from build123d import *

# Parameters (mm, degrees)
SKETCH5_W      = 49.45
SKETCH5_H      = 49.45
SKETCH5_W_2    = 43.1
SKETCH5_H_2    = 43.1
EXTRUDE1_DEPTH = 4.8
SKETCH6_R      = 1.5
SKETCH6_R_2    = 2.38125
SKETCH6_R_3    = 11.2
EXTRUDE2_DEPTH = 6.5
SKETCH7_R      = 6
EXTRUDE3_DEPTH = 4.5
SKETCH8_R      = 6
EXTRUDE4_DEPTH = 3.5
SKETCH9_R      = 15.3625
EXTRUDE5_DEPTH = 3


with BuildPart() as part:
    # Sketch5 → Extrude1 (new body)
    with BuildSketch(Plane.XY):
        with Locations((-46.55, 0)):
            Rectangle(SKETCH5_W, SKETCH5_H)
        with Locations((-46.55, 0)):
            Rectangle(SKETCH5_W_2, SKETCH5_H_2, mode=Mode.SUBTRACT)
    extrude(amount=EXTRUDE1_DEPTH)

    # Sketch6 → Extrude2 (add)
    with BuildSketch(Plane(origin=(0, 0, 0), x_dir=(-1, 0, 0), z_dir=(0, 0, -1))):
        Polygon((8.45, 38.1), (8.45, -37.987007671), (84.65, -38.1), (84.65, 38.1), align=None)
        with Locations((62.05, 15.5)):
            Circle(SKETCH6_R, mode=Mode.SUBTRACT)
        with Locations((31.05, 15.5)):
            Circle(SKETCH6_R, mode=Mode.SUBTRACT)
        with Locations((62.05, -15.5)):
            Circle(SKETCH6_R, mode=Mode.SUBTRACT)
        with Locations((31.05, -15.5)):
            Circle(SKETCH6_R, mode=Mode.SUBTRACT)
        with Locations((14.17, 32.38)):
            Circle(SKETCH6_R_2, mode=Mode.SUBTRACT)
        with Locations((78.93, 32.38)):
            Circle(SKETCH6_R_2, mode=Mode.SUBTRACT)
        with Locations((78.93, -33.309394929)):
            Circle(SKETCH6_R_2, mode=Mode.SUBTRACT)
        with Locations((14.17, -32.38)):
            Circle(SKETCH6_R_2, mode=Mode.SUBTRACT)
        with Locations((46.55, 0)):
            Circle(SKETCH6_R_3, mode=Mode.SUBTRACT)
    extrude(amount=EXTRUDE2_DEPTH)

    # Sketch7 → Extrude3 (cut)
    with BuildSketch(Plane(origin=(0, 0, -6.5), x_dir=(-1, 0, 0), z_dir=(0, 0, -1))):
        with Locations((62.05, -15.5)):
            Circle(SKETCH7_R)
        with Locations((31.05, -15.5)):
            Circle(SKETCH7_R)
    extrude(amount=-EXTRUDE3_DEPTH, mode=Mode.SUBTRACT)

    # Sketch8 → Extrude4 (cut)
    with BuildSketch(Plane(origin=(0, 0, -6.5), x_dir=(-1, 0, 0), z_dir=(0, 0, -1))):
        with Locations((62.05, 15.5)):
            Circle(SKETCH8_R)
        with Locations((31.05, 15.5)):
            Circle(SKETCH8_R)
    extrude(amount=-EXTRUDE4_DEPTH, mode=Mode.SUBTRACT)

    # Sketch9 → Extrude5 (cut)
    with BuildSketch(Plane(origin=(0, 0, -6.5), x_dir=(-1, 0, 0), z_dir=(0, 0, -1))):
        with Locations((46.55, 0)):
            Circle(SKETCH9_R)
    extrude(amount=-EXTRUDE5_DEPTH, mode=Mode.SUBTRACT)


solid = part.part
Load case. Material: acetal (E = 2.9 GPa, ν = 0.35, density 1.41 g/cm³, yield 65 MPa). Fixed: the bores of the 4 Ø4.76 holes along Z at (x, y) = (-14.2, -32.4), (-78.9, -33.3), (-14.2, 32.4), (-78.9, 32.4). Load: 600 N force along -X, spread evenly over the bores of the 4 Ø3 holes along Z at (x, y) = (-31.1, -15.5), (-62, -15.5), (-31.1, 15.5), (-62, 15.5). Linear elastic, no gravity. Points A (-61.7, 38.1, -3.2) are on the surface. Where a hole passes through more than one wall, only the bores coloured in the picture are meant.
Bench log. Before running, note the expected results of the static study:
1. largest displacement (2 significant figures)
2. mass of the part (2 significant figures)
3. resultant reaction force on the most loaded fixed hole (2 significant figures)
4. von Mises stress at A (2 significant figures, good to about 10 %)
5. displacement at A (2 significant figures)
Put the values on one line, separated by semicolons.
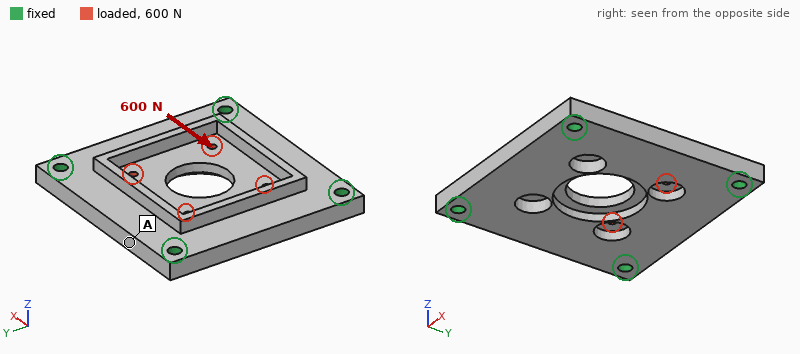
28 µm; 49 g; 180 N; 0.85 MPa; 6.6 µm
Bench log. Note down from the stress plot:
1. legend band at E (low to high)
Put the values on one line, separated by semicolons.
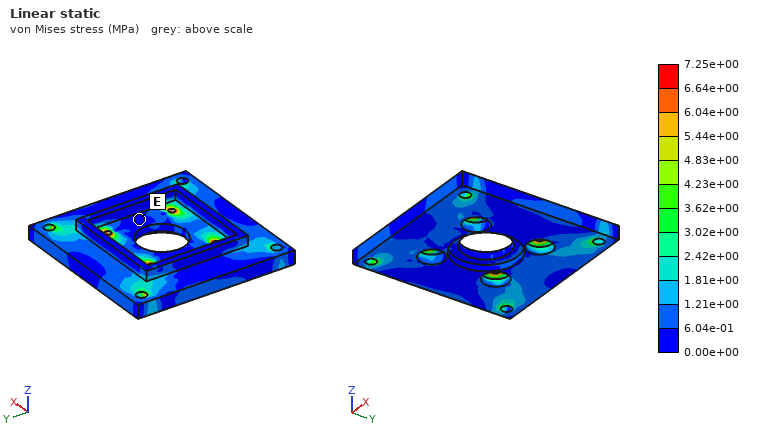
0.00e+00 to 6.04e-01 MPa
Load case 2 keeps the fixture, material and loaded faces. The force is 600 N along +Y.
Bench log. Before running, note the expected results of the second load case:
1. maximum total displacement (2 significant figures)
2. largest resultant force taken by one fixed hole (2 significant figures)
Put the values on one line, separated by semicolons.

28 µm; 170 N
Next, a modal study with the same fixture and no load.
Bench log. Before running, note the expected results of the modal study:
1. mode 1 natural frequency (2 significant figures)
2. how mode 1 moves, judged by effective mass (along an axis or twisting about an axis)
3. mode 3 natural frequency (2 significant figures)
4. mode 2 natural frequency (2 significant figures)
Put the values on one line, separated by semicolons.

1600 Hz; along Z; 2400 Hz; 2400 Hz
